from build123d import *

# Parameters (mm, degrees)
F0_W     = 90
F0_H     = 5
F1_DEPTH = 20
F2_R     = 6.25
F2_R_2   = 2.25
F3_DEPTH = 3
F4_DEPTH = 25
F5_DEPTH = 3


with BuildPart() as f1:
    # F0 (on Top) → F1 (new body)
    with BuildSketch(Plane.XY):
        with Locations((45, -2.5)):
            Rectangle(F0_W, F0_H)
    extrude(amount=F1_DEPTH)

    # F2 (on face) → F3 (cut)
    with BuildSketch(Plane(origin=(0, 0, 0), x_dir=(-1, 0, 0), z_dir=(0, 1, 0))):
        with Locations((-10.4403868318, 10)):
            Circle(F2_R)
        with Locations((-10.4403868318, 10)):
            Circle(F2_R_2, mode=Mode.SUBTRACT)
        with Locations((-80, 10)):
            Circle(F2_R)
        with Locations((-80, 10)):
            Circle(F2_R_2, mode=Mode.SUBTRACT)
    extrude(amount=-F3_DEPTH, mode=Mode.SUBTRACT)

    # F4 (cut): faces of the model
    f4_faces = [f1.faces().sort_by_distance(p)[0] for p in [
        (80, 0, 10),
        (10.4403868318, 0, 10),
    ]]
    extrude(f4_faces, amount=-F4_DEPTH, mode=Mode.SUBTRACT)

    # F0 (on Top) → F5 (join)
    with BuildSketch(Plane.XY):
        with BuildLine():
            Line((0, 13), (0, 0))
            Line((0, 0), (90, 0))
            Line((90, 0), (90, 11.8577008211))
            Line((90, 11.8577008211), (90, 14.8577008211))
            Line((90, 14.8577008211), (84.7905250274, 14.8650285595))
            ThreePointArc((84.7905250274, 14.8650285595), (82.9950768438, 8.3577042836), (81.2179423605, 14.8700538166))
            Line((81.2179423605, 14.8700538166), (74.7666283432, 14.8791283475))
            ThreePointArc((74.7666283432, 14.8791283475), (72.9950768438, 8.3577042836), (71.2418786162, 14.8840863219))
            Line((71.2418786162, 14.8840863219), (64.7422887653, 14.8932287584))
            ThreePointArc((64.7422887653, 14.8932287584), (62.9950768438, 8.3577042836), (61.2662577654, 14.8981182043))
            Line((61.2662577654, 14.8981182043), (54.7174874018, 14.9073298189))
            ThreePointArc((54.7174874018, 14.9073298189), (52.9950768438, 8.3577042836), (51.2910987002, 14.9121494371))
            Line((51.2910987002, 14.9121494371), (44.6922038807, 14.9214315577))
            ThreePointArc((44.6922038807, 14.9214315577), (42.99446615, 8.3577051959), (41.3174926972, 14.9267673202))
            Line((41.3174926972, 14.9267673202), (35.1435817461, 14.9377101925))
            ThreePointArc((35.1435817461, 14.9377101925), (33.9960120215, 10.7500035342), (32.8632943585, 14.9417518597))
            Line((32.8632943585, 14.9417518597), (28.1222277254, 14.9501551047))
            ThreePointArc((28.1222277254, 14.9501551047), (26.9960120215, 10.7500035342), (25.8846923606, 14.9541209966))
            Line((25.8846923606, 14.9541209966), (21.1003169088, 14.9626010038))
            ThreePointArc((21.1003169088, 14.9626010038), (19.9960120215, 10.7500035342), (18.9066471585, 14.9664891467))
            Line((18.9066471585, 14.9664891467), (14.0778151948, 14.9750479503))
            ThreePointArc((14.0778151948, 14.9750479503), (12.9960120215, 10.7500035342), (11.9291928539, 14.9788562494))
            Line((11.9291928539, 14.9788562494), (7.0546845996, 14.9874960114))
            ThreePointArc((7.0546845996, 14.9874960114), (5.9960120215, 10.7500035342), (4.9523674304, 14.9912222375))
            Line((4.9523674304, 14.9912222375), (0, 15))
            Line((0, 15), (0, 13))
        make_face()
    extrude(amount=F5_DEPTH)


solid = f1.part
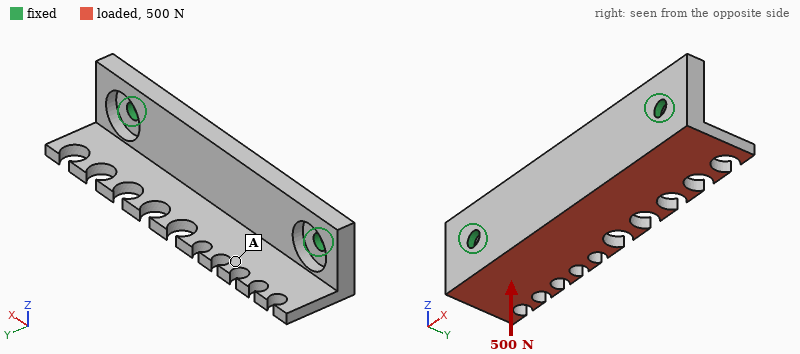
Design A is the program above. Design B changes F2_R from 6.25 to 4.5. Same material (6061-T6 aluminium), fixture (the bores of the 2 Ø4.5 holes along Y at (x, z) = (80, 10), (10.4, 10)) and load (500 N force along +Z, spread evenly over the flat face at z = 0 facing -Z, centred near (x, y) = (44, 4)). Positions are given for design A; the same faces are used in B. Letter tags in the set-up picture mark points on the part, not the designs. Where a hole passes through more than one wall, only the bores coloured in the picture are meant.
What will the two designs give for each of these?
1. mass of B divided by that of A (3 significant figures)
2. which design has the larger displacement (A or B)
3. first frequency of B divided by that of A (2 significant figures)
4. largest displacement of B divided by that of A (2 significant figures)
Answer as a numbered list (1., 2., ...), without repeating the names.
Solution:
1. 1.03
2. A
3. 1.1
4. 0.85
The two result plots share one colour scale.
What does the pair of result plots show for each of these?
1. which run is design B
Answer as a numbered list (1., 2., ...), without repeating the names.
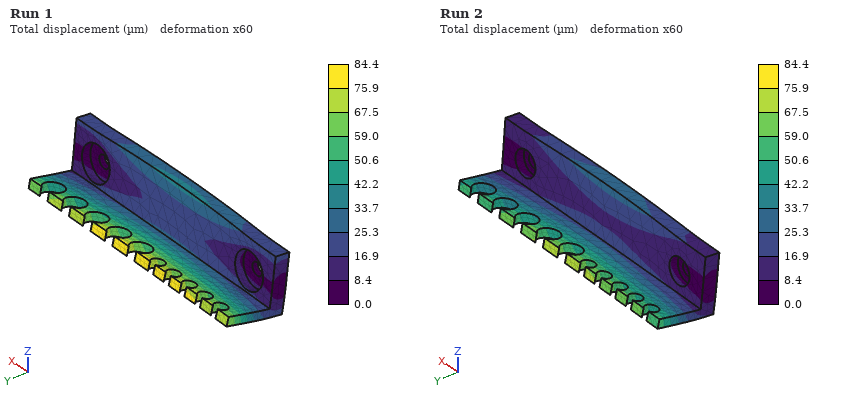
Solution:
1. Run 2
